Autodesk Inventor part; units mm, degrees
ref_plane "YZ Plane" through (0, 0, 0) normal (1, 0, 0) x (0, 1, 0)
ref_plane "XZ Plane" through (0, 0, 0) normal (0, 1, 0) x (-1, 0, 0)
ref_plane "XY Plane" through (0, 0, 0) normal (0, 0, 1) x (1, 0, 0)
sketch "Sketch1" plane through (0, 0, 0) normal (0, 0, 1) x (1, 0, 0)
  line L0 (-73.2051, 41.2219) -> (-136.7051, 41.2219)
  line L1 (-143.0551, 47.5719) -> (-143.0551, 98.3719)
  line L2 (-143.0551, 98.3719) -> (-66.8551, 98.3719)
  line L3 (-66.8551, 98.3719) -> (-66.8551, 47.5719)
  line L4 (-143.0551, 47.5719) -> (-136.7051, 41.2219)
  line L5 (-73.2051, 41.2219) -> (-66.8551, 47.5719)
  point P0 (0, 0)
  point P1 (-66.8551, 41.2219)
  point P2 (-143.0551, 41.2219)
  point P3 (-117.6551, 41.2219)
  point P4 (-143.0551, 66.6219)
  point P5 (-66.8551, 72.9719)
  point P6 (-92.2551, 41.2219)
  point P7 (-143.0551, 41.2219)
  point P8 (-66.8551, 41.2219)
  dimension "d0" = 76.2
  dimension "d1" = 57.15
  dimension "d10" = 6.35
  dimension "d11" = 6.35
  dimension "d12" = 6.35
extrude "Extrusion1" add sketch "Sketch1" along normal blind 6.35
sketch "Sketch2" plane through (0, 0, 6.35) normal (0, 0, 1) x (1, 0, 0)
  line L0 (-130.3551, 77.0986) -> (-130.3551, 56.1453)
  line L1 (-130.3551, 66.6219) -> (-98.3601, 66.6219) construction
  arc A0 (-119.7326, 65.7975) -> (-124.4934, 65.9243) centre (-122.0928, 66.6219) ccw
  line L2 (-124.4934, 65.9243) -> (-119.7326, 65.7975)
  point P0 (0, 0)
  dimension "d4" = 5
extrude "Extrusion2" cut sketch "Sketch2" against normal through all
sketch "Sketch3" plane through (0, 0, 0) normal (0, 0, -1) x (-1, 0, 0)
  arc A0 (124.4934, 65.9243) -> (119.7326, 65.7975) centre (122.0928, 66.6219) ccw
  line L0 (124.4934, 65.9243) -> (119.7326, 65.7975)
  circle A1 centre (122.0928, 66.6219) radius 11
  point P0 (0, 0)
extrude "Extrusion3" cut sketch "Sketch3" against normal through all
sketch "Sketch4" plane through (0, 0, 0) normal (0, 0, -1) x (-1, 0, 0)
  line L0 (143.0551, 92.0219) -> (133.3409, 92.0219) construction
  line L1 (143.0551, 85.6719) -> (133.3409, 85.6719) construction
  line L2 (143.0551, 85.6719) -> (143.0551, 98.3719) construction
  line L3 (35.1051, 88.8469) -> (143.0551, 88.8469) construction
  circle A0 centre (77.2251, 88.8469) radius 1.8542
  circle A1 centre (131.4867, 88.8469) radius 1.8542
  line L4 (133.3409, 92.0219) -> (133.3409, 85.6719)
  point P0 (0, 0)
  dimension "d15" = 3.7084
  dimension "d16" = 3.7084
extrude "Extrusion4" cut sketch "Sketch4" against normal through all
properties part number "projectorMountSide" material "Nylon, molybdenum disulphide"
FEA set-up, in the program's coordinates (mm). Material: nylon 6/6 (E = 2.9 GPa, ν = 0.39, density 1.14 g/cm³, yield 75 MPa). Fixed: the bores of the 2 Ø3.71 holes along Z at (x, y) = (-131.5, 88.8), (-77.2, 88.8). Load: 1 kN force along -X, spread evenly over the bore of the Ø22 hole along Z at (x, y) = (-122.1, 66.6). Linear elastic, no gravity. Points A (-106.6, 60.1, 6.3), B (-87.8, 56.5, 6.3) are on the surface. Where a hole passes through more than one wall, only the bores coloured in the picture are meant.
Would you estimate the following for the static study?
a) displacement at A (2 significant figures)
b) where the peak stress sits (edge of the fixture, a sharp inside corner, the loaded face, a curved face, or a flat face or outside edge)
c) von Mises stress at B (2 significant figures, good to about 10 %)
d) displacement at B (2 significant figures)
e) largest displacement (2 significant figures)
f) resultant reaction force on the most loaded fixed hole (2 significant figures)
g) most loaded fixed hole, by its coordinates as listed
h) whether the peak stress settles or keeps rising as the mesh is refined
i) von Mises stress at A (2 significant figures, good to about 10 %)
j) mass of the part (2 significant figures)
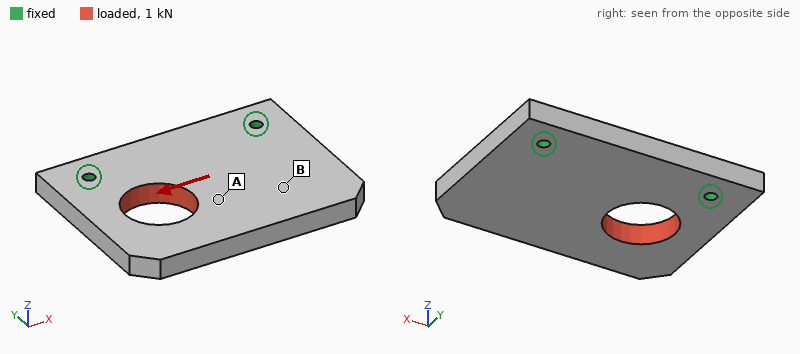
0.11 mm
edge of the fixture
1.8 MPa
0.10 mm
0.17 mm
700 N
(-131.5, 88.8)
keeps rising
4.9 MPa
28 g
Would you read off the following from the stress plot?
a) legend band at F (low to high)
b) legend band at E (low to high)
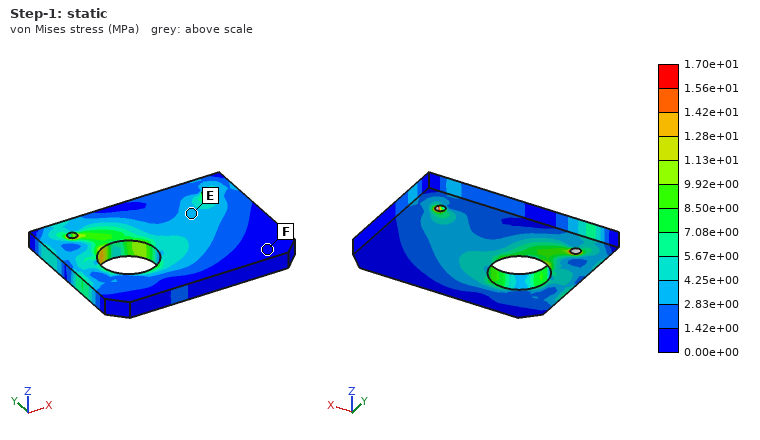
0.00e+00 to 1.42e+00 MPa
2.83e+00 to 4.25e+00 MPa
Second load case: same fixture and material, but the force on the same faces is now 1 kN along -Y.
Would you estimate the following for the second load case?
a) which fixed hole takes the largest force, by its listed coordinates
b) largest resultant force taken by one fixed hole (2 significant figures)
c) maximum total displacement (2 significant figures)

(-131.5, 88.8)
830 N
0.11 mm
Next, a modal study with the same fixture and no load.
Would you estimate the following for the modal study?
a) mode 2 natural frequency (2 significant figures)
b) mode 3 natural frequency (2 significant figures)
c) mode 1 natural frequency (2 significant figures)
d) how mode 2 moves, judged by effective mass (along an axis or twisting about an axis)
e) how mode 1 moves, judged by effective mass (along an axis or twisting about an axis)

1200 Hz
2300 Hz
570 Hz
twisting about Y
along Z
